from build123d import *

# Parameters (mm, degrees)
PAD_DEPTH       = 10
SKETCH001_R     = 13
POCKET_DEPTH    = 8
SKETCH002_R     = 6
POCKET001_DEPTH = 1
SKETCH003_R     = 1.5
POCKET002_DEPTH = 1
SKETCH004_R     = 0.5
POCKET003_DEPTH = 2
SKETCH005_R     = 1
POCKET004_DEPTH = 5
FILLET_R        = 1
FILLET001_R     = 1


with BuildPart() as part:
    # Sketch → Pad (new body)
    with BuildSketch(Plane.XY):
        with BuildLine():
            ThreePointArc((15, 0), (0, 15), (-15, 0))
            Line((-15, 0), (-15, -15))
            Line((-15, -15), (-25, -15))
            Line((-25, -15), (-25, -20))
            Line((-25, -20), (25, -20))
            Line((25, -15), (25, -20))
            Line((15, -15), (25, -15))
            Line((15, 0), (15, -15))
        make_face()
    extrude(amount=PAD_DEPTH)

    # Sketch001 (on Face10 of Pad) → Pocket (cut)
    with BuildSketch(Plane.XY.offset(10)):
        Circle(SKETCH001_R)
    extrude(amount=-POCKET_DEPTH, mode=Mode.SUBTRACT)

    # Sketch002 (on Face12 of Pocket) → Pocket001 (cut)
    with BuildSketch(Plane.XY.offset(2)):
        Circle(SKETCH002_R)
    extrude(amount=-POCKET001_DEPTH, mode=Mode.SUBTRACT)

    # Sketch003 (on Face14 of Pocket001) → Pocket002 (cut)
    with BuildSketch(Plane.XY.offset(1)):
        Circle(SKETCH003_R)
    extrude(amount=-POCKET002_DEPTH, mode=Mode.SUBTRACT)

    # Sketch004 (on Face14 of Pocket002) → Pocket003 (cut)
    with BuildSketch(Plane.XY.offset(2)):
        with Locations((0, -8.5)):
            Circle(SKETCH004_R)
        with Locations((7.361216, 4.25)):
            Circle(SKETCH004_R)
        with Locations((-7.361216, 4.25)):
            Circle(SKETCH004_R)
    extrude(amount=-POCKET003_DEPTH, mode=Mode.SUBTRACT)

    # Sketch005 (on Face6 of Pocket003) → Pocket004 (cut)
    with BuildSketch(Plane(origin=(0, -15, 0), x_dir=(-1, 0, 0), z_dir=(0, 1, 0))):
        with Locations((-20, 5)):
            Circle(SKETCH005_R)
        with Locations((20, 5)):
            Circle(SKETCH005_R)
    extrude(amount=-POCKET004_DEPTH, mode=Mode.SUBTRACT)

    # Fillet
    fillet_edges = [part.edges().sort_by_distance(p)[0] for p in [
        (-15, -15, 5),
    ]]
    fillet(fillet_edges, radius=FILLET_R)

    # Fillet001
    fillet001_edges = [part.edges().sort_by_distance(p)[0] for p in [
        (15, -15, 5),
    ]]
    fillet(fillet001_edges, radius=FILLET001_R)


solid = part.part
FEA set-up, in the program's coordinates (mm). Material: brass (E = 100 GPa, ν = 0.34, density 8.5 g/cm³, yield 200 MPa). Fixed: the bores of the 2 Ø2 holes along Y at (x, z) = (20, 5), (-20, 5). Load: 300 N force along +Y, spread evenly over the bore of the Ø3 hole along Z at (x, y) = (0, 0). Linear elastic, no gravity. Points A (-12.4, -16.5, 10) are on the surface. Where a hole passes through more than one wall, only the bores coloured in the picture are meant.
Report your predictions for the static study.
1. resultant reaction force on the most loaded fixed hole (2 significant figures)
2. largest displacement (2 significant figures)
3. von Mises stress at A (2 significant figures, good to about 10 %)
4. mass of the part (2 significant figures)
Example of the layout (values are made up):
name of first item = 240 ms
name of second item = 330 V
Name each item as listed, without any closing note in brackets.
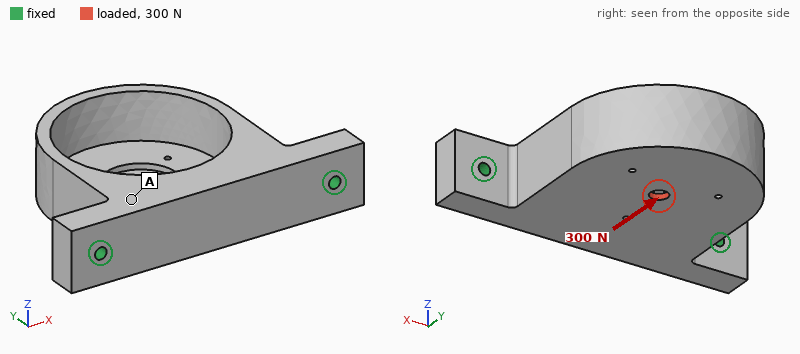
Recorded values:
resultant reaction force on the most loaded fixed hole = 170 N
largest displacement = 18 µm
von Mises stress at A = 4.4 MPa
mass of the part = 52 g
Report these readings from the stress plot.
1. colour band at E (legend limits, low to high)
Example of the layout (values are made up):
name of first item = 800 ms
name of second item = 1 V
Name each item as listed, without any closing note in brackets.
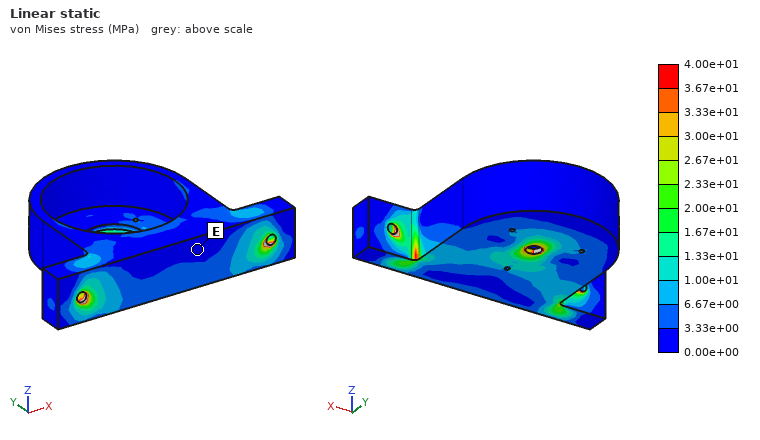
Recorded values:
colour band at E = 0.00e+00 to 3.33e+00 MPa
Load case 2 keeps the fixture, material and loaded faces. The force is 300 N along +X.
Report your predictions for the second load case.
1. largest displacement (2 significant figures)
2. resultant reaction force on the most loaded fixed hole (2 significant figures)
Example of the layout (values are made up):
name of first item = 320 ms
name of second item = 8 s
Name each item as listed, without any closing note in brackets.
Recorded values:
largest displacement = 6.4 µm
resultant reaction force on the most loaded fixed hole = 210 N
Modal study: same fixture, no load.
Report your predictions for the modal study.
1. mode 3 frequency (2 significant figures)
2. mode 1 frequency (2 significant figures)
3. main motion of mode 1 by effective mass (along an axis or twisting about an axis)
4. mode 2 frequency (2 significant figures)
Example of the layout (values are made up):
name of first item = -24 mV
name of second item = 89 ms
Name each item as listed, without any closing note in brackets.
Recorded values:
mode 3 frequency = 9200 Hz
mode 1 frequency = 2500 Hz
main motion of mode 1 by effective mass = along Z
mode 2 frequency = 6000 Hz
